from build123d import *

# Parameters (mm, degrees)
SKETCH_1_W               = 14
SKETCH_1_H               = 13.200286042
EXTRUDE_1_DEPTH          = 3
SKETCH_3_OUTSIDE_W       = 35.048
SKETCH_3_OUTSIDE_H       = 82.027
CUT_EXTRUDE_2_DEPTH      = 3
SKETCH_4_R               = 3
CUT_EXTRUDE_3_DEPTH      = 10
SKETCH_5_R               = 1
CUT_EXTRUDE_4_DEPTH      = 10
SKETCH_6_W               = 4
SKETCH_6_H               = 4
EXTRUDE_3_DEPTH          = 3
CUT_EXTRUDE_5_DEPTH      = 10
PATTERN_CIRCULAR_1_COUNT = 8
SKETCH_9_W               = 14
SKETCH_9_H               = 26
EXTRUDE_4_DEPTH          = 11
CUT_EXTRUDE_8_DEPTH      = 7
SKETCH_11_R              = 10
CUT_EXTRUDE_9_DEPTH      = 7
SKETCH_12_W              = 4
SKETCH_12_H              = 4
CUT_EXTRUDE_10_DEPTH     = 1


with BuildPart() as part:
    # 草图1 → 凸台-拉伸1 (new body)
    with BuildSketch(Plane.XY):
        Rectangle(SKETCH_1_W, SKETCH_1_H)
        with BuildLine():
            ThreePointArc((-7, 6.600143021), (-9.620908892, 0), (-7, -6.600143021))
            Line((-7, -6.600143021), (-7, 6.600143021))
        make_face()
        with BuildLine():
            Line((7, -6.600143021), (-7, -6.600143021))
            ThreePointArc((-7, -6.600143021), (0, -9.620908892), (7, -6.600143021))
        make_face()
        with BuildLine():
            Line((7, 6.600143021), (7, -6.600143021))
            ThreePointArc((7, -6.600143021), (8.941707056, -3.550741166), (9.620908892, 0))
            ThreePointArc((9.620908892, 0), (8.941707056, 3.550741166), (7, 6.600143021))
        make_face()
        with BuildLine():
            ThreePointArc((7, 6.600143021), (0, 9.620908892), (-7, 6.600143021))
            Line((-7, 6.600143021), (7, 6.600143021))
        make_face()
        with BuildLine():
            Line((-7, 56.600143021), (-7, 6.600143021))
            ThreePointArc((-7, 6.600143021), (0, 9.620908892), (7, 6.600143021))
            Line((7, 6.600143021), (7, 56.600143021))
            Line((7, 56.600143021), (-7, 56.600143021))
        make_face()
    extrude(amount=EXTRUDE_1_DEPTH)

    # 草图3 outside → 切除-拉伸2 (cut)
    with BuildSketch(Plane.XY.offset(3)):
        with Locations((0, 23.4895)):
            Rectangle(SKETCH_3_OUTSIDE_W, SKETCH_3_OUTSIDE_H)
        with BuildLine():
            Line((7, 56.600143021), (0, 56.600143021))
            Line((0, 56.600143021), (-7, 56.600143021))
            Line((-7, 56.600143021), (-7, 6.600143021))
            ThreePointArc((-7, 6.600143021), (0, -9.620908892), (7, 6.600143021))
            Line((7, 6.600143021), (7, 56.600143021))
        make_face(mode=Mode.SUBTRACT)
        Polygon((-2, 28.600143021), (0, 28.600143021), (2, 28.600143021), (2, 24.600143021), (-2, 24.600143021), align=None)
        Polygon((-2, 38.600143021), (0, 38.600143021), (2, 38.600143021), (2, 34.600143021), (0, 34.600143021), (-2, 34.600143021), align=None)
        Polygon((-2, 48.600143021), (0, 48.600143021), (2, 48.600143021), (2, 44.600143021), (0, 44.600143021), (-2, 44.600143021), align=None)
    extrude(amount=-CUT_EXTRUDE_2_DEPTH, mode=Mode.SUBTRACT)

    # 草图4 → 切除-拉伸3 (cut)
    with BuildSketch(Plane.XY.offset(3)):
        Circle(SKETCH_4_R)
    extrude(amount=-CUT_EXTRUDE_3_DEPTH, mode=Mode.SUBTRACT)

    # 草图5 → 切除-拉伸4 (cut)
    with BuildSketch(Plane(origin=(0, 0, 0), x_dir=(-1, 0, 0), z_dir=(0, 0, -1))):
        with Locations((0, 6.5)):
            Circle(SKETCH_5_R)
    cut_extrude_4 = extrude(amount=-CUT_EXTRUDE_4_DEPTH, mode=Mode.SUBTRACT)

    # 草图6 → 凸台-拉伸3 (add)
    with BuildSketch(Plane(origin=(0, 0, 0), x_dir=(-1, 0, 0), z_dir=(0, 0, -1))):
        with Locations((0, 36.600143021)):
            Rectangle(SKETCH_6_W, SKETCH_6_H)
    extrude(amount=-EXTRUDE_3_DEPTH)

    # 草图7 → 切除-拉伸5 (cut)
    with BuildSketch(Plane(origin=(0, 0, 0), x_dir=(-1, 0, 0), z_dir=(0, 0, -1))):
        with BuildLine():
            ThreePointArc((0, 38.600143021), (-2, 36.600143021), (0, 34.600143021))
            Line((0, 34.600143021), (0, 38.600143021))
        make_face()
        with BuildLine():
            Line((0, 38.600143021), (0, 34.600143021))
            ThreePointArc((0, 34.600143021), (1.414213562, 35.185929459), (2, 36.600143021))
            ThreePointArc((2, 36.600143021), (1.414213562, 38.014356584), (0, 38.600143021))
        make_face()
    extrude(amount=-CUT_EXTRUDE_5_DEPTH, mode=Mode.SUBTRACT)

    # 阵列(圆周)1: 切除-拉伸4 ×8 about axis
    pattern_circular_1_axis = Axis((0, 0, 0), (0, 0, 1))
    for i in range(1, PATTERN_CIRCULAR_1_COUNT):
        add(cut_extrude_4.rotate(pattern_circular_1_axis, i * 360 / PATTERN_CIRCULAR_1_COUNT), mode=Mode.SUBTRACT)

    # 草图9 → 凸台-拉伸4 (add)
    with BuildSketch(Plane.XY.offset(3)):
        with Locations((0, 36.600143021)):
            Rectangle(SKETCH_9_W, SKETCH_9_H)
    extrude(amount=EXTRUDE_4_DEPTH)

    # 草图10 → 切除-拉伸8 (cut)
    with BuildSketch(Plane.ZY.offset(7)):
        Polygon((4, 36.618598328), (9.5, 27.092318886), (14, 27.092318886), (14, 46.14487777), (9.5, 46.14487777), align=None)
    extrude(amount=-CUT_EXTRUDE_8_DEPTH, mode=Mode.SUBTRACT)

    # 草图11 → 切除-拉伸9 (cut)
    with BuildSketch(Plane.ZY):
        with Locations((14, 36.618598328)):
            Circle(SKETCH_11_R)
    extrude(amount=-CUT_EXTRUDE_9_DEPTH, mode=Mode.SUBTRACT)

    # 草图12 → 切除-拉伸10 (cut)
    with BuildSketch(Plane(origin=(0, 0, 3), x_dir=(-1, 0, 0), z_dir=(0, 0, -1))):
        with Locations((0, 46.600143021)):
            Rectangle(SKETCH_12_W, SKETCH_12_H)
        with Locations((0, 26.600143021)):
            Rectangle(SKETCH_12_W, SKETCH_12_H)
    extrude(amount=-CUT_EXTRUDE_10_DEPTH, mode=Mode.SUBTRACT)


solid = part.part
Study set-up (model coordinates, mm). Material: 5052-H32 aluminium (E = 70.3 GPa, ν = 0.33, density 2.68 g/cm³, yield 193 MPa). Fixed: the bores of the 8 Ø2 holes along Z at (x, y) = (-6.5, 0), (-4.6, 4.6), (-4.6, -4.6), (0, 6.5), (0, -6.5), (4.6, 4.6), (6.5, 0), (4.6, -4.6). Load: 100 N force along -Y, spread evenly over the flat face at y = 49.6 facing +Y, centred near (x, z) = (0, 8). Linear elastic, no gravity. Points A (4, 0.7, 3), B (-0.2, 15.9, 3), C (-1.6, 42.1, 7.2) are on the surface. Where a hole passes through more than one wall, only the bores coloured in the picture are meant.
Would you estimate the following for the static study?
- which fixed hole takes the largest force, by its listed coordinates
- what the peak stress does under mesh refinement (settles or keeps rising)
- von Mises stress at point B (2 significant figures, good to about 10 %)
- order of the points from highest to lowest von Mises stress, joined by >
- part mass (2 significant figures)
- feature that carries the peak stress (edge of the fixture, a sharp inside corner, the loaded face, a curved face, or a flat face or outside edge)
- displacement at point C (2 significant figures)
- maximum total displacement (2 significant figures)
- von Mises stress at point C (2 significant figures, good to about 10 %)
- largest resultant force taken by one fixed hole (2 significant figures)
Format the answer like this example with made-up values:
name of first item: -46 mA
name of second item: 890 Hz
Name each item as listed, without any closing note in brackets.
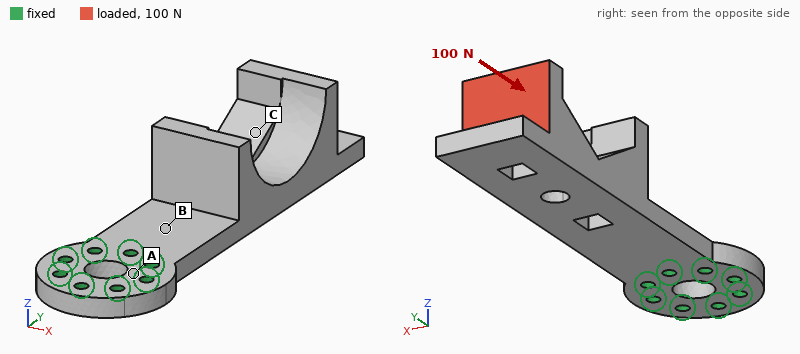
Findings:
which fixed hole takes the largest force, by its listed coordinates: (0, 6.5)
what the peak stress does under mesh refinement: keeps rising
von Mises stress at point B: 33 MPa
order of the points from highest to lowest von Mises stress, joined by >: B > C > A
part mass: 12 g
feature that carries the peak stress: edge of the fixture
displacement at point C: 0.16 mm
maximum total displacement: 0.26 mm
von Mises stress at point C: 6.8 MPa
largest resultant force taken by one fixed hole: 74 N
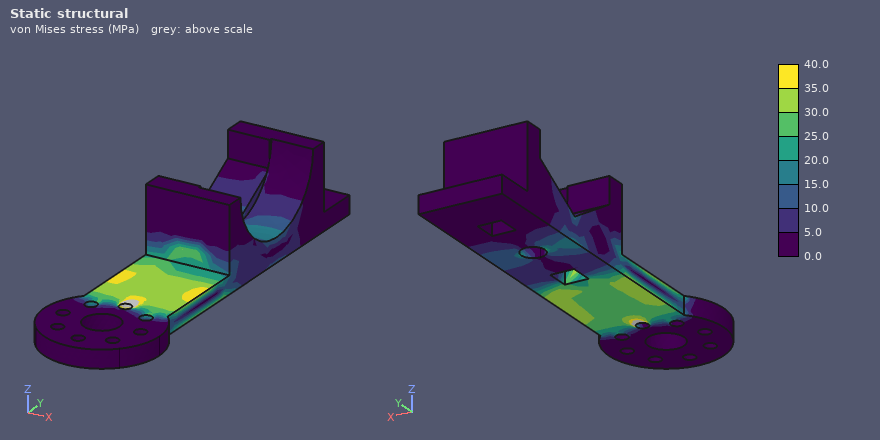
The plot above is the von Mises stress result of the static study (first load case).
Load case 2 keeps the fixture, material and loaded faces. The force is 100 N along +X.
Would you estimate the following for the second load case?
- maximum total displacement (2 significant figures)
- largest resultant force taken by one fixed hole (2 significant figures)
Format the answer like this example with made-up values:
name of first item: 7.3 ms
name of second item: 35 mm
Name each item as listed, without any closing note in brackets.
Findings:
maximum total displacement: 0.11 mm
largest resultant force taken by one fixed hole: 350 N
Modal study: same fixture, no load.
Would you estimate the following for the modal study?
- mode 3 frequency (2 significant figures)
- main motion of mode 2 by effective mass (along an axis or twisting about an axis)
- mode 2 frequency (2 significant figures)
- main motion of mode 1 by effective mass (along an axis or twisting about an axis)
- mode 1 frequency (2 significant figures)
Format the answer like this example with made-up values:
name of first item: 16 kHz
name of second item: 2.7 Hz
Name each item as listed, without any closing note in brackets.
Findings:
mode 3 frequency: 4400 Hz
main motion of mode 2 by effective mass: along X
mode 2 frequency: 2800 Hz
main motion of mode 1 by effective mass: along Z
mode 1 frequency: 740 Hz
